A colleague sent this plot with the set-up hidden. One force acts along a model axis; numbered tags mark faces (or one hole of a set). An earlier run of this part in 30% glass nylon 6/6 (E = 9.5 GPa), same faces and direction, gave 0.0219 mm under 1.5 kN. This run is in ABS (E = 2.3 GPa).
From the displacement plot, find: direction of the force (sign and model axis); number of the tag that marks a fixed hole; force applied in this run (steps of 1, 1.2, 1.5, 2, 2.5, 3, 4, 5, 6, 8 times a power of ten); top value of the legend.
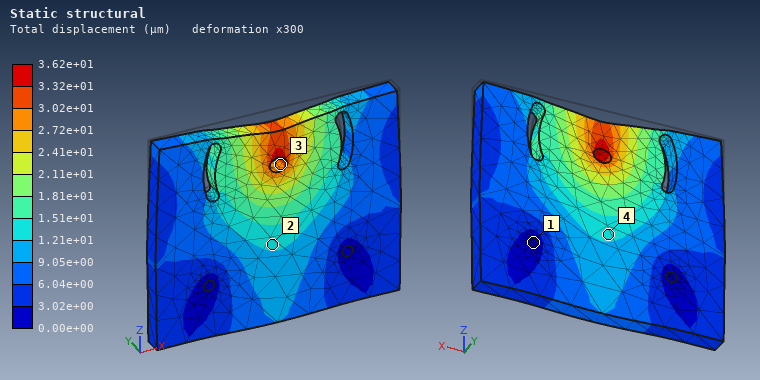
-Z
1
600 N
3.62e+01 µm
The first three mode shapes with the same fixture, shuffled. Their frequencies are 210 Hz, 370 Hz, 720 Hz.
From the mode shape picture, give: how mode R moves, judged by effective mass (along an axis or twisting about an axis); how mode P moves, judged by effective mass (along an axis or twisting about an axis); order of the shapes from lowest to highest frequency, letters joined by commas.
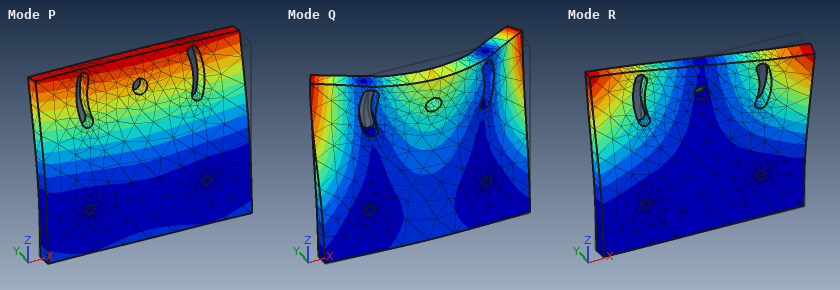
twisting about Z
along Y
P, R, Q
